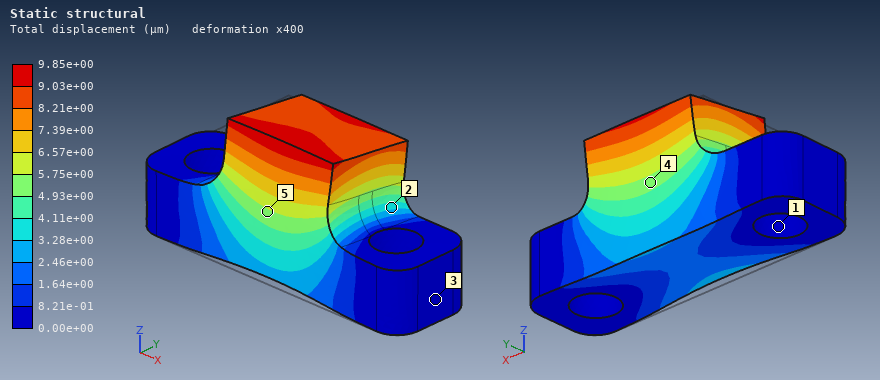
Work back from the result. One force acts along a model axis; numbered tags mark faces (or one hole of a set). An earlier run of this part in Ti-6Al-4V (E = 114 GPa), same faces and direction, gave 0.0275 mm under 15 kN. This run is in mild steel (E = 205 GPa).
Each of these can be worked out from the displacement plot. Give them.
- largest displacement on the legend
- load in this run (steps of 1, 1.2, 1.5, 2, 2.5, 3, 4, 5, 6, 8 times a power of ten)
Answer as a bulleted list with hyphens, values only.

- 9.85e+00 µm
- 10 kN
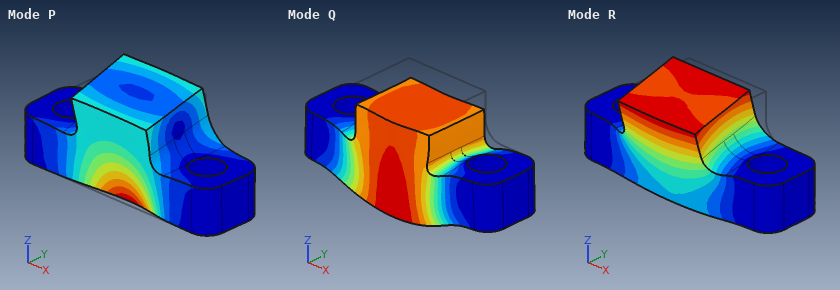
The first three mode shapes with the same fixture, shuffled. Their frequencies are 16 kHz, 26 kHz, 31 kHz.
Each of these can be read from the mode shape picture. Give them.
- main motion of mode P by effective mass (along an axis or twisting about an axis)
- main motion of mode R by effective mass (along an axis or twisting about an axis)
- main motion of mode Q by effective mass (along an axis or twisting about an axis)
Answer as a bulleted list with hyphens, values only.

- along Y
- along Y
- along Z
